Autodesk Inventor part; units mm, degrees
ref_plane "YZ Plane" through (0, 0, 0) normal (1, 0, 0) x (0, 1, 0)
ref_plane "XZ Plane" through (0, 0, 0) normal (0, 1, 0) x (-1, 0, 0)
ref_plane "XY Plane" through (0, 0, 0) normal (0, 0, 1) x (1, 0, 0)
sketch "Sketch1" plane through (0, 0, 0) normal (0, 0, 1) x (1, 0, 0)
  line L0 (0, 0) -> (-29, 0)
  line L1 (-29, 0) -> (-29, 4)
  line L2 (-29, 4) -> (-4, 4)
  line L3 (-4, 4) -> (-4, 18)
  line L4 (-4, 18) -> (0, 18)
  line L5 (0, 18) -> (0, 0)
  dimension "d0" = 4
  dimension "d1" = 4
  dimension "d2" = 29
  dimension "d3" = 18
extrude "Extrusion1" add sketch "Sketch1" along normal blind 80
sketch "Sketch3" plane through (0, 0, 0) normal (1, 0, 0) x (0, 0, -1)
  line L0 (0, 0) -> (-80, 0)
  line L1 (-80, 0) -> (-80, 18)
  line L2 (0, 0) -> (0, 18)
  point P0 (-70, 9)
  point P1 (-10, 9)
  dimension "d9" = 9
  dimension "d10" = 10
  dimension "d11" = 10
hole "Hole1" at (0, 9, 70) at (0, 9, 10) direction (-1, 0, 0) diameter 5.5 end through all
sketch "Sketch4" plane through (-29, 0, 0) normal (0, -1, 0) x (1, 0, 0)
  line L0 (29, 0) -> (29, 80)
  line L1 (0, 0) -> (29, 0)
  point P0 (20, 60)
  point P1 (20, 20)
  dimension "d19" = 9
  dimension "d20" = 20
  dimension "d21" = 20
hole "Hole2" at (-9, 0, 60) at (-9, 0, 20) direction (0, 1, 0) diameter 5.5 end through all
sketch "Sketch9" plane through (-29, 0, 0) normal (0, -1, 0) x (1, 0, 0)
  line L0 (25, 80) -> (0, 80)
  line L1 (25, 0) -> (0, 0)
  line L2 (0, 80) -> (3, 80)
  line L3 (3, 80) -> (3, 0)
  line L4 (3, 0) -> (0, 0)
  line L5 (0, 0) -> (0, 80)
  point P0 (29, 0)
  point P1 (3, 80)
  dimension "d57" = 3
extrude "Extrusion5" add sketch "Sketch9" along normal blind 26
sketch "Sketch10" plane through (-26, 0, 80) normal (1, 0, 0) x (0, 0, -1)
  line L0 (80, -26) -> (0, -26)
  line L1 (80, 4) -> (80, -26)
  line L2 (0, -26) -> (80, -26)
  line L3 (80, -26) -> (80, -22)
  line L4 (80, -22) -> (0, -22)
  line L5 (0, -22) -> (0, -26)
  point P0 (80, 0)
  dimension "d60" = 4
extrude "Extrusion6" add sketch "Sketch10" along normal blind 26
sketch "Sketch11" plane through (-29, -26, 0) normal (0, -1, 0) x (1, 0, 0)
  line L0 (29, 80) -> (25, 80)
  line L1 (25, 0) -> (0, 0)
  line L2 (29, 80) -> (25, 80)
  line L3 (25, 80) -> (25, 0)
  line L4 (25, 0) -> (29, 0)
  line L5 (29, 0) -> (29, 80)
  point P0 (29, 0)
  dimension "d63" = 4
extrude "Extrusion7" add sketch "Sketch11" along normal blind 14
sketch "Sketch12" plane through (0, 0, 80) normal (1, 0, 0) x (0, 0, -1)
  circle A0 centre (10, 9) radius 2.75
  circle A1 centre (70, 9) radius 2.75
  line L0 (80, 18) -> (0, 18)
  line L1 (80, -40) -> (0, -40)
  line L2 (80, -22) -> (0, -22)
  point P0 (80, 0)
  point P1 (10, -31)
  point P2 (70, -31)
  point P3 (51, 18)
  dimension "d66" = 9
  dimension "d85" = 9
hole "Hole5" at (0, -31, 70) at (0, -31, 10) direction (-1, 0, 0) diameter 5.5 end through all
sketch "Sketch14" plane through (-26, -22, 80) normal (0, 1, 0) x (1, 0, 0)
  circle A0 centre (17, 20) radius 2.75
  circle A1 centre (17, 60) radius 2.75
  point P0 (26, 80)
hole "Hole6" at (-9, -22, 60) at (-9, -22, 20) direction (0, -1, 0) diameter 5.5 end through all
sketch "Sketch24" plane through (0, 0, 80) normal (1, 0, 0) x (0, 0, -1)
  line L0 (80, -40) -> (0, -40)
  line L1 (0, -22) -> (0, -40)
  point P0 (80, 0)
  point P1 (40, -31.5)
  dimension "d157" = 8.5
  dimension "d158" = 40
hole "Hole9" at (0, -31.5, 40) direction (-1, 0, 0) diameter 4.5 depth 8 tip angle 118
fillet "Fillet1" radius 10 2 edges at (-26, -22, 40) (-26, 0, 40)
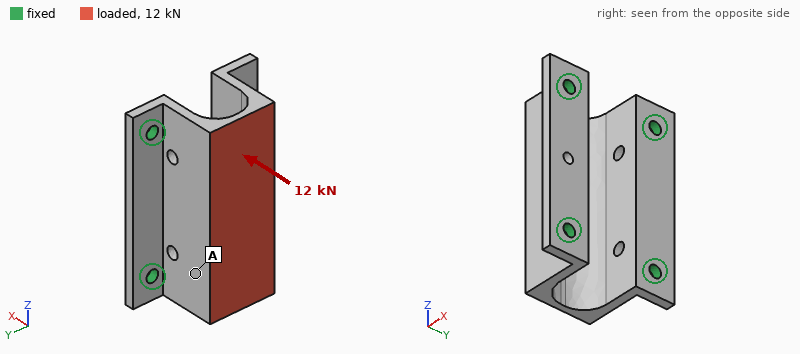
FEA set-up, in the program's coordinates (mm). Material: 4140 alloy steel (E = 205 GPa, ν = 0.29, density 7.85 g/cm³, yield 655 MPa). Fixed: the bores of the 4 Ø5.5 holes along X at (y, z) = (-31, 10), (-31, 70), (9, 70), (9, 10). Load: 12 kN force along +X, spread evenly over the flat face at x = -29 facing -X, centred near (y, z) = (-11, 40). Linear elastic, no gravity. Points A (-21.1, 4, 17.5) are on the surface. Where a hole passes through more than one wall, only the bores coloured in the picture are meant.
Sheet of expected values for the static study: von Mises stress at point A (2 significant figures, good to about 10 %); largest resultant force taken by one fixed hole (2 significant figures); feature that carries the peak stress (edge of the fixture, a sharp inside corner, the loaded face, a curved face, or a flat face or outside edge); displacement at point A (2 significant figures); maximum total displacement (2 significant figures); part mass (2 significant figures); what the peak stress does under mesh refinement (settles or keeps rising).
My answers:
21 MPa
3.2 kN
edge of the fixture
11 µm
19 µm
280 g
keeps rising
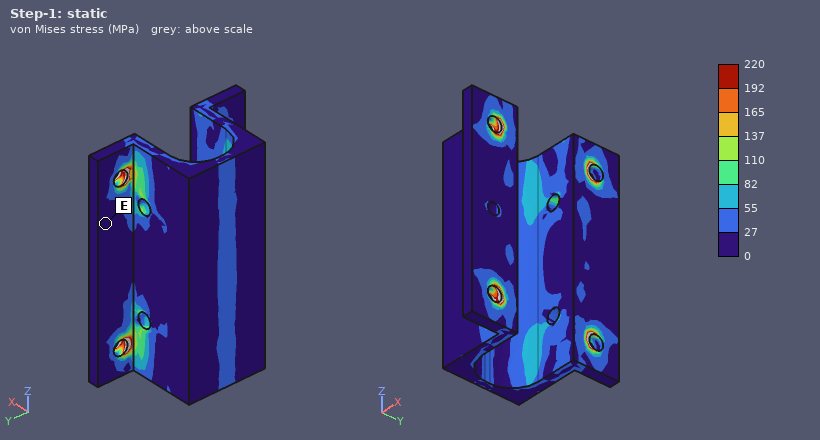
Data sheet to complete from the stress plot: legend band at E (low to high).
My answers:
0 to 27 MPa
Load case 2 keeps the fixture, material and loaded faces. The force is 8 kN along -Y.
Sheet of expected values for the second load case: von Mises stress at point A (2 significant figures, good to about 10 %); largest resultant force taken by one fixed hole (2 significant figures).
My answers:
78 MPa
3.5 kN
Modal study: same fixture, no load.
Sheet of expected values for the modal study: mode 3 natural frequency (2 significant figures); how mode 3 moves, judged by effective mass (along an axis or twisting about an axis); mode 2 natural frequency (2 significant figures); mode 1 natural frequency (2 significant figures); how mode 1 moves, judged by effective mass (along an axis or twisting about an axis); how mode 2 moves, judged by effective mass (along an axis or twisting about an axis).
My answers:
9600 Hz
along X
7000 Hz
4800 Hz
along Y
twisting about X
